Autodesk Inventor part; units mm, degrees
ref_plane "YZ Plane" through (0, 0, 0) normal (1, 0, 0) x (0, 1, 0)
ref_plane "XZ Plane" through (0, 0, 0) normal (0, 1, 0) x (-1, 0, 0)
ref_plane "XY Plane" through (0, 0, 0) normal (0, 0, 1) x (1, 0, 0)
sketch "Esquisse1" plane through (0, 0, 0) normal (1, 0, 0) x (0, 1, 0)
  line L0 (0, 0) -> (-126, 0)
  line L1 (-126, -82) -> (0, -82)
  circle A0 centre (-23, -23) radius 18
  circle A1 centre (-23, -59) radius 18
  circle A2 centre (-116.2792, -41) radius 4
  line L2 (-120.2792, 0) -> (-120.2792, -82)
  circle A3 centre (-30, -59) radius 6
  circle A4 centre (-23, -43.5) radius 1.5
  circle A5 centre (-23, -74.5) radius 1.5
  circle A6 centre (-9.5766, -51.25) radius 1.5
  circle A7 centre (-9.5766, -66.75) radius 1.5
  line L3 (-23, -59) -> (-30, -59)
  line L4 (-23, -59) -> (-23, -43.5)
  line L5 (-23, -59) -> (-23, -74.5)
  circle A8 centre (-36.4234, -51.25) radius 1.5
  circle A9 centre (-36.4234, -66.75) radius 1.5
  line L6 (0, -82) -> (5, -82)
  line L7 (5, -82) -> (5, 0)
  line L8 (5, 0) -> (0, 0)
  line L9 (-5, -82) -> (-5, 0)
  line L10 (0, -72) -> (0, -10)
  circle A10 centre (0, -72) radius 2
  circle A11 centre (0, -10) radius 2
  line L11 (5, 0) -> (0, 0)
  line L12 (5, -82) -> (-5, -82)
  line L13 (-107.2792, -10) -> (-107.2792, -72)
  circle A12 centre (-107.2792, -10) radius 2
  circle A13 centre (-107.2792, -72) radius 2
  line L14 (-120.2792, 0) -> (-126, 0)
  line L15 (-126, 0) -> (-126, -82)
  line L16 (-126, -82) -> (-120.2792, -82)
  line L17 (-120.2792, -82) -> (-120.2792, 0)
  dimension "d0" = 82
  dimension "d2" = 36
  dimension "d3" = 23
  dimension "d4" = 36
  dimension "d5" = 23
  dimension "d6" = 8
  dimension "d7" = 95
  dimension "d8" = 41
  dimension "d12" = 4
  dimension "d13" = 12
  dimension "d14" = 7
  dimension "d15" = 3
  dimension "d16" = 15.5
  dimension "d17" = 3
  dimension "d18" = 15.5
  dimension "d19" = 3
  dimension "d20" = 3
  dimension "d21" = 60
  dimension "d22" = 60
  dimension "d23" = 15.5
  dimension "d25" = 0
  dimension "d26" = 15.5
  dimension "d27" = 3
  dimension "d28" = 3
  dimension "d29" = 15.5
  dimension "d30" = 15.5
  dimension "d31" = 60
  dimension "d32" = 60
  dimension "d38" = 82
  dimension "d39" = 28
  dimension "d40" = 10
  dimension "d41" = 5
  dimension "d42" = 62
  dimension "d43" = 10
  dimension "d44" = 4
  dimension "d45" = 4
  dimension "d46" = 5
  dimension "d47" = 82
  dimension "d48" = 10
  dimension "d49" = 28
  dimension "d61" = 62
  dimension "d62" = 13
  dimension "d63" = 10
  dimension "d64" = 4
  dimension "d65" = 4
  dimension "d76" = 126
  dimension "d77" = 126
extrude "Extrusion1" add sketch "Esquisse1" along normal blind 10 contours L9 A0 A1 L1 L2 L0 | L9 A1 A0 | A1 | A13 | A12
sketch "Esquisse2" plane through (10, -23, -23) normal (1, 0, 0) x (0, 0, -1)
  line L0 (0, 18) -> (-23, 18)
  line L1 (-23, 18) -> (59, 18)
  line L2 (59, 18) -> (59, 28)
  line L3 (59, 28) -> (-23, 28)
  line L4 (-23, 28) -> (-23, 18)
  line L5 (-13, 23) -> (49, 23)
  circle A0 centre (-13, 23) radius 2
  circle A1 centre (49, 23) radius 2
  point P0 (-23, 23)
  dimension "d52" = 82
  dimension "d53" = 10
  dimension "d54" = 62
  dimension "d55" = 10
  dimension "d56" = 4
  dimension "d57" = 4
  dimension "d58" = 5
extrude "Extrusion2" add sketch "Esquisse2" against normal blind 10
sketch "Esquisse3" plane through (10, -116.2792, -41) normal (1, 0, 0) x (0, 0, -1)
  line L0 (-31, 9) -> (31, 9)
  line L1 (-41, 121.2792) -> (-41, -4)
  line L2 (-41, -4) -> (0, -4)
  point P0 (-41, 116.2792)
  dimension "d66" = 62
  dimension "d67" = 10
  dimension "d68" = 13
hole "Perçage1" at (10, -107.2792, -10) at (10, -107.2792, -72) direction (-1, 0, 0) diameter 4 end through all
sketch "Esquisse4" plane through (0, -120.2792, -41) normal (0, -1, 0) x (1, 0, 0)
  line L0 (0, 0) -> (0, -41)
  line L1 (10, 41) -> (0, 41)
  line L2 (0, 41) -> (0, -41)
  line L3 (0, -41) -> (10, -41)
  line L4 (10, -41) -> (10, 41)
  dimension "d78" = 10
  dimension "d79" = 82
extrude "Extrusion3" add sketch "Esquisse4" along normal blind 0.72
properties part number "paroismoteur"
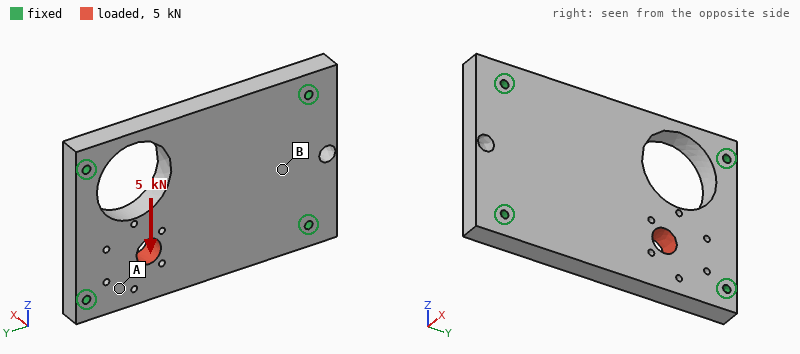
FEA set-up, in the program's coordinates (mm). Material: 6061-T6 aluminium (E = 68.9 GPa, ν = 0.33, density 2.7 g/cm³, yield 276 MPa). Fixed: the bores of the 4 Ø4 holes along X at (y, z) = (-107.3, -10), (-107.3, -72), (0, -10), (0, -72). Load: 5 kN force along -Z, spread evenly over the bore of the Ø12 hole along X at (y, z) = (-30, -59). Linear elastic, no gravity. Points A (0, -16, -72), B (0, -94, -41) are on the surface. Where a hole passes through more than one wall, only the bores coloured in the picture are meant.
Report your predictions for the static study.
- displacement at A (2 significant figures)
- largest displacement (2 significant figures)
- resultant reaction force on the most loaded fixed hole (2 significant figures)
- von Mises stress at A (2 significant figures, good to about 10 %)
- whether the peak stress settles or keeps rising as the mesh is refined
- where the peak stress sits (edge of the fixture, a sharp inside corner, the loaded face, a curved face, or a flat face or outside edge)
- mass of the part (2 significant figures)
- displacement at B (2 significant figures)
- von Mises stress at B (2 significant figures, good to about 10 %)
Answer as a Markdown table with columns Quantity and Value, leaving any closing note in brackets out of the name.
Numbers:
| Quantity | Value |
|---|---|
| displacement at A | 9.5 µm |
| largest displacement | 17 µm |
| resultant reaction force on the most loaded fixed hole | 2.1 kN |
| von Mises stress at A | 9.8 MPa |
| whether the peak stress settles or keeps rising as the mesh is refined | keeps rising |
| where the peak stress sits | edge of the fixture |
| mass of the part | 240 g |
| displacement at B | 2.6 µm |
| von Mises stress at B | 4.8 MPa |
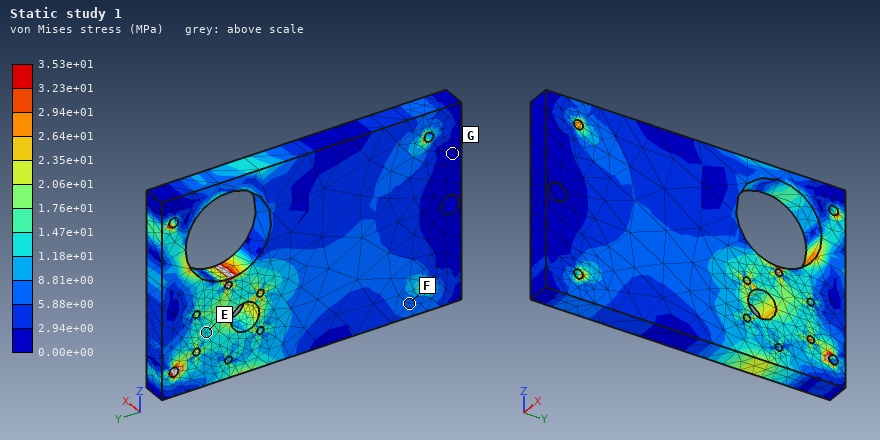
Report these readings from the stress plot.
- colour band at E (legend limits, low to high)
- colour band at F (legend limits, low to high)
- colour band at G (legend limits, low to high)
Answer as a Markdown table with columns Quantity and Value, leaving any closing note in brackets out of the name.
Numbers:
| Quantity | Value |
|---|---|
| colour band at E | 1.18e+01 to 1.47e+01 MPa |
| colour band at F | 5.88e+00 to 8.81e+00 MPa |
| colour band at G | 0.00e+00 to 2.94e+00 MPa |
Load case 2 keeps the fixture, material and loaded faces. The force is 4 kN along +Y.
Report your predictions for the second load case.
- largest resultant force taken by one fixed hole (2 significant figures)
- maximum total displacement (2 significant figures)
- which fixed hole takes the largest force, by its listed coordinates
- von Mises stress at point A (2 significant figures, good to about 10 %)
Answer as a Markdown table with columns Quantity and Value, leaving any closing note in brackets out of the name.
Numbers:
| Quantity | Value |
|---|---|
| largest resultant force taken by one fixed hole | 1.9 kN |
| maximum total displacement | 6.9 µm |
| which fixed hole takes the largest force, by its listed coordinates | (0, -72) |
| von Mises stress at point A | 9.7 MPa |
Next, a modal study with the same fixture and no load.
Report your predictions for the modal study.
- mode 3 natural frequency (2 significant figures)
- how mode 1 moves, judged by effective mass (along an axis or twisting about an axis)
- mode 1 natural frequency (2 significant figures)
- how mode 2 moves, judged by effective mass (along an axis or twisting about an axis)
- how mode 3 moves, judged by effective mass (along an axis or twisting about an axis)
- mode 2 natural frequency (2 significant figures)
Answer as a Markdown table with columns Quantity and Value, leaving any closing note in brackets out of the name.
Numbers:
| Quantity | Value |
|---|---|
| mode 3 natural frequency | 8500 Hz |
| how mode 1 moves, judged by effective mass | along X |
| mode 1 natural frequency | 3300 Hz |
| how mode 2 moves, judged by effective mass | twisting about Y |
| how mode 3 moves, judged by effective mass | twisting about Z |
| mode 2 natural frequency | 4900 Hz |
